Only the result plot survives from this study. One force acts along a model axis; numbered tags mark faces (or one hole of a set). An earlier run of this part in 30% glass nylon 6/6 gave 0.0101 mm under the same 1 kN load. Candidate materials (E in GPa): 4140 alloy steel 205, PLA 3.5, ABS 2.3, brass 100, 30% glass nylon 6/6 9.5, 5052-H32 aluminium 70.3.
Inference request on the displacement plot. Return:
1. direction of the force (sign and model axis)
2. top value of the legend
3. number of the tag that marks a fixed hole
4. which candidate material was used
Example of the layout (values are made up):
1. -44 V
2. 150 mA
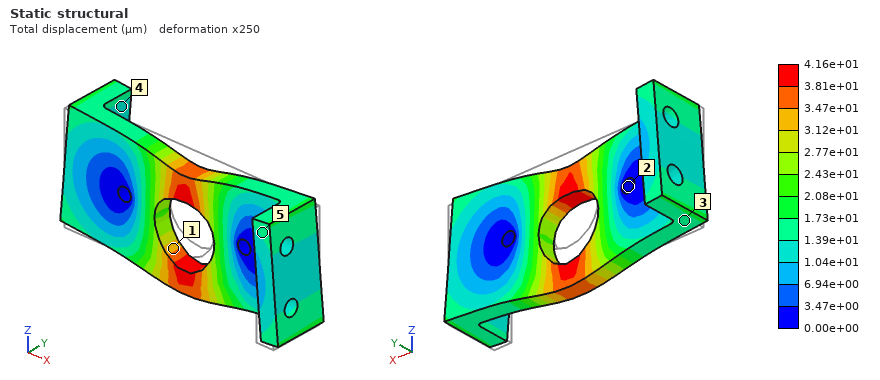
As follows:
1. -Z
2. 4.16e+01 µm
3. 2
4. ABS
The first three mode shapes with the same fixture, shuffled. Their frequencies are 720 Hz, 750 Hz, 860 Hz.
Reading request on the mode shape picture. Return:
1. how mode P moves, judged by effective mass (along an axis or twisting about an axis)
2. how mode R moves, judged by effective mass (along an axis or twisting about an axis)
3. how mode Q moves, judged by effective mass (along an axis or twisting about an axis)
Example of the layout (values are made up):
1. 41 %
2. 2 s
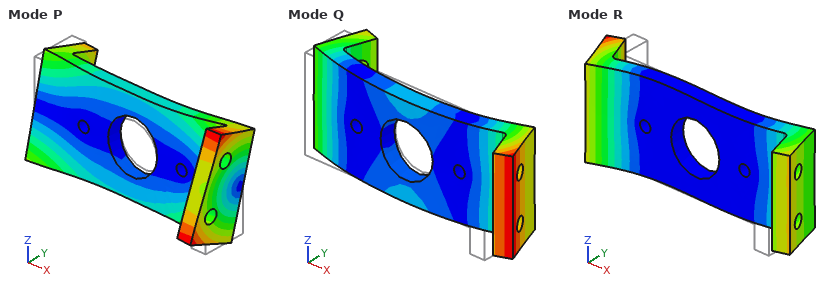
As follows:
1. twisting about X
2. twisting about Z
3. along Y
